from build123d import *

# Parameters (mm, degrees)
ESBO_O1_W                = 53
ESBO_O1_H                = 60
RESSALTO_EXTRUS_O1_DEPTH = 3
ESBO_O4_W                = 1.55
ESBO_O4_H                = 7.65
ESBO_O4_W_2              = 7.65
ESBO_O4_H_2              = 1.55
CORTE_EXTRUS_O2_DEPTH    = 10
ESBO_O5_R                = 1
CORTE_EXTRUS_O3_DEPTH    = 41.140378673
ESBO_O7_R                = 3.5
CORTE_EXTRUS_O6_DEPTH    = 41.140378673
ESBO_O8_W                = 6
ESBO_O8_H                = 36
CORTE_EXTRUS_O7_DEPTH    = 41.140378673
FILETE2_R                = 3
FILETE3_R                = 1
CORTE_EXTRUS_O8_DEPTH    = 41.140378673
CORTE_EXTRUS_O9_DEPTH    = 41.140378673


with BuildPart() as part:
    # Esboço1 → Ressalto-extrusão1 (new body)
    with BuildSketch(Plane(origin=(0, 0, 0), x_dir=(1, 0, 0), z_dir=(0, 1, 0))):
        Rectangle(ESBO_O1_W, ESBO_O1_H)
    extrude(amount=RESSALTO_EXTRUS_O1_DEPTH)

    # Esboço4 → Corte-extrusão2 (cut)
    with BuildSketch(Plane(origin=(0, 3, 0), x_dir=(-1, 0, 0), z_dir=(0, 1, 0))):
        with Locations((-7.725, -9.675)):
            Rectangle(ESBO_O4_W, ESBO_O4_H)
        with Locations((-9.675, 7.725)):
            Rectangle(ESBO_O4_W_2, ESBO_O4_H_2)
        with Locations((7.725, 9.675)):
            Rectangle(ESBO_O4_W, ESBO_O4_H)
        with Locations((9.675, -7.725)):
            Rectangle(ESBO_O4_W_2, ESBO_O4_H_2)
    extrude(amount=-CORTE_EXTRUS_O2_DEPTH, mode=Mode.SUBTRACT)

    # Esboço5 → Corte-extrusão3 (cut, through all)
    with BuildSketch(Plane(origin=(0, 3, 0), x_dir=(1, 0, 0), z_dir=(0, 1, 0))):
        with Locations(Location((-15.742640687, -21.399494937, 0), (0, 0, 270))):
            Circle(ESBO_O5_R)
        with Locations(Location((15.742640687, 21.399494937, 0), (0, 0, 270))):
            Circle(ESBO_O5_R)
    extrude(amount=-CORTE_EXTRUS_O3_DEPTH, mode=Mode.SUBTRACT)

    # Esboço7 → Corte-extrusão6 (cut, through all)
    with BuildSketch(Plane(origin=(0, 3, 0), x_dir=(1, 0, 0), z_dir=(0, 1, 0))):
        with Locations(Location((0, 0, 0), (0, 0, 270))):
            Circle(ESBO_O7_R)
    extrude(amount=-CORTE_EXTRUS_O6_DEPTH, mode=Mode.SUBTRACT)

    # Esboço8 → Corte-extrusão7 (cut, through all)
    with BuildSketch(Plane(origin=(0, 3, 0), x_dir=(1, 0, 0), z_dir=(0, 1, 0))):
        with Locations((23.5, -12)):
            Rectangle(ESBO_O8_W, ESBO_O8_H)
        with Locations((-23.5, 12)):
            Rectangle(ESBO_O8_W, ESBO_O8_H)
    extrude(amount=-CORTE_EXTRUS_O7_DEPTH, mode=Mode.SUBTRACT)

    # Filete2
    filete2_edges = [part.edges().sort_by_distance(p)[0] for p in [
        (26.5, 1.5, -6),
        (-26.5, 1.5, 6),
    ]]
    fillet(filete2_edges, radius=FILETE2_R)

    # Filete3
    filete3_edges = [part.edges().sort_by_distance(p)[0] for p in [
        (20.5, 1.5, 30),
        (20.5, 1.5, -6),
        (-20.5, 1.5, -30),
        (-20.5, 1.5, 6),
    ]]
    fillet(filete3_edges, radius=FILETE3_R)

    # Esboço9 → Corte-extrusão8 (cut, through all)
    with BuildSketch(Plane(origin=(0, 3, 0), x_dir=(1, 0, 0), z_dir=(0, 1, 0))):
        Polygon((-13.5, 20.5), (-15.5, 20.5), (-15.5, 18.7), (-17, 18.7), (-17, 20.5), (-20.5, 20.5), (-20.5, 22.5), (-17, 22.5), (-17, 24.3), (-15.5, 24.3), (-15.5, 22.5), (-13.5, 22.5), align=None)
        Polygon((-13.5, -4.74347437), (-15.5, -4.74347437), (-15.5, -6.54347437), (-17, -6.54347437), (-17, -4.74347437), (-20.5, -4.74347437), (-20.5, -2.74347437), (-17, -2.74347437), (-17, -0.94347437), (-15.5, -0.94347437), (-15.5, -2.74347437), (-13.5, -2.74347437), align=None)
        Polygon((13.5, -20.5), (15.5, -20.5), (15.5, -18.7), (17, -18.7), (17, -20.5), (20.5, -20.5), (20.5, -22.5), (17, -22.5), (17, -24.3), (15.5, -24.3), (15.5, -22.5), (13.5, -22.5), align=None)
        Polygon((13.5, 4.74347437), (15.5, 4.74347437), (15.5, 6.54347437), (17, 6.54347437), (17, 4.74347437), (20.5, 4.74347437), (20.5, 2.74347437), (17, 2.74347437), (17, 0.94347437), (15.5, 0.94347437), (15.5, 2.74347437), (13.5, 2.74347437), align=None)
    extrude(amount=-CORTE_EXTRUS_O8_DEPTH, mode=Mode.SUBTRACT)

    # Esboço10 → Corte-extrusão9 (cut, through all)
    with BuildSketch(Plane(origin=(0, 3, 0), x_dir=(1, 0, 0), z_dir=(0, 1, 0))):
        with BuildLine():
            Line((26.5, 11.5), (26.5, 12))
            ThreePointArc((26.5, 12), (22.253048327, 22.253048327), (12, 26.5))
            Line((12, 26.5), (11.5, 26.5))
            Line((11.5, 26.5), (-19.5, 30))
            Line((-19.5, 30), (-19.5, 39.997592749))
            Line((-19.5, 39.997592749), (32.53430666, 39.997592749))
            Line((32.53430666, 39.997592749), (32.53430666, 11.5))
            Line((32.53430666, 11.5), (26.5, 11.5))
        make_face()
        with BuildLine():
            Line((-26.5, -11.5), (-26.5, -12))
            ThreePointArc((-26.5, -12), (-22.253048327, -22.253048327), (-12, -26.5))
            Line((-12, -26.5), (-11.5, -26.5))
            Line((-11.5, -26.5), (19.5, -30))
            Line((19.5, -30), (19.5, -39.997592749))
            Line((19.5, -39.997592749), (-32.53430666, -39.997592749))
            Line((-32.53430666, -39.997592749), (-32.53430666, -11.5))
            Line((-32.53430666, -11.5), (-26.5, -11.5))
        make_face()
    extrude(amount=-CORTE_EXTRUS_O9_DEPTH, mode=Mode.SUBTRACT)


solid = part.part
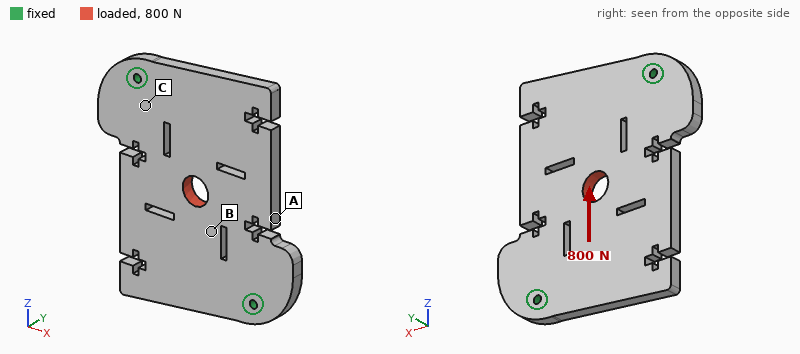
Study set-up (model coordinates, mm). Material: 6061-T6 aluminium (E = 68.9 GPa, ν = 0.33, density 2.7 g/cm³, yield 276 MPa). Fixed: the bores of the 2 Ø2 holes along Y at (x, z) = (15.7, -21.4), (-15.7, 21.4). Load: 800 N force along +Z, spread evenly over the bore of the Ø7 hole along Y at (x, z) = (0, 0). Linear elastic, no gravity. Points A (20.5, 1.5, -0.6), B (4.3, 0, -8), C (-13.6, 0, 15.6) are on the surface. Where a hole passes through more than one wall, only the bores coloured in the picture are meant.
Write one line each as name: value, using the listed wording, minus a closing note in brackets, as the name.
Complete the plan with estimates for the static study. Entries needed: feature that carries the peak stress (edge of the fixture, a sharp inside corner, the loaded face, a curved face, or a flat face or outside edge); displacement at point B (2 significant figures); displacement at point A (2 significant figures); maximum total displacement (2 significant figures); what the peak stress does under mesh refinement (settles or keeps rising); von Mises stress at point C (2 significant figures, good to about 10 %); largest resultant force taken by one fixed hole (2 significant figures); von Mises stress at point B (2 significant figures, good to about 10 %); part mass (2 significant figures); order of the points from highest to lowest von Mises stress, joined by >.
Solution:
feature that carries the peak stress: edge of the fixture
displacement at point B: 7.1 µm
displacement at point A: 8.8 µm
maximum total displacement: 9.5 µm
what the peak stress does under mesh refinement: keeps rising
von Mises stress at point C: 15 MPa
largest resultant force taken by one fixed hole: 400 N
von Mises stress at point B: 8.5 MPa
part mass: 18 g
order of the points from highest to lowest von Mises stress, joined by >: C > B > A
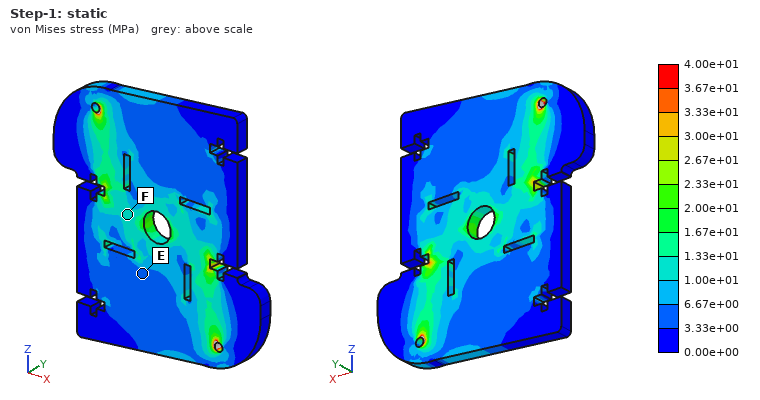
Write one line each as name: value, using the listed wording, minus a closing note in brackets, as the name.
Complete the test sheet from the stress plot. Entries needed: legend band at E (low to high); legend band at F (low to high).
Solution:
legend band at E: 3.33e+00 to 6.67e+00 MPa
legend band at F: 1.00e+01 to 1.33e+01 MPa
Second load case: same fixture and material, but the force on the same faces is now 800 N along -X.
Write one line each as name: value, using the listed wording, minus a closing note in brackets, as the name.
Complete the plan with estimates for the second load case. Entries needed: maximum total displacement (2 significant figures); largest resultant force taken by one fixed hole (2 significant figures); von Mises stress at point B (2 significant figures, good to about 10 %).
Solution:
maximum total displacement: 14 µm
largest resultant force taken by one fixed hole: 400 N
von Mises stress at point B: 13 MPa
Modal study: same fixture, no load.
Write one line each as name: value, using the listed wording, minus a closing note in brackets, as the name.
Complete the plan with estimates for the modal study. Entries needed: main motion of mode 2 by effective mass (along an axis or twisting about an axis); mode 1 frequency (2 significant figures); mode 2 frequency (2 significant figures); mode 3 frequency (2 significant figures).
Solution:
main motion of mode 2 by effective mass: along Y
mode 1 frequency: 2000 Hz
mode 2 frequency: 2600 Hz
mode 3 frequency: 5300 Hz
